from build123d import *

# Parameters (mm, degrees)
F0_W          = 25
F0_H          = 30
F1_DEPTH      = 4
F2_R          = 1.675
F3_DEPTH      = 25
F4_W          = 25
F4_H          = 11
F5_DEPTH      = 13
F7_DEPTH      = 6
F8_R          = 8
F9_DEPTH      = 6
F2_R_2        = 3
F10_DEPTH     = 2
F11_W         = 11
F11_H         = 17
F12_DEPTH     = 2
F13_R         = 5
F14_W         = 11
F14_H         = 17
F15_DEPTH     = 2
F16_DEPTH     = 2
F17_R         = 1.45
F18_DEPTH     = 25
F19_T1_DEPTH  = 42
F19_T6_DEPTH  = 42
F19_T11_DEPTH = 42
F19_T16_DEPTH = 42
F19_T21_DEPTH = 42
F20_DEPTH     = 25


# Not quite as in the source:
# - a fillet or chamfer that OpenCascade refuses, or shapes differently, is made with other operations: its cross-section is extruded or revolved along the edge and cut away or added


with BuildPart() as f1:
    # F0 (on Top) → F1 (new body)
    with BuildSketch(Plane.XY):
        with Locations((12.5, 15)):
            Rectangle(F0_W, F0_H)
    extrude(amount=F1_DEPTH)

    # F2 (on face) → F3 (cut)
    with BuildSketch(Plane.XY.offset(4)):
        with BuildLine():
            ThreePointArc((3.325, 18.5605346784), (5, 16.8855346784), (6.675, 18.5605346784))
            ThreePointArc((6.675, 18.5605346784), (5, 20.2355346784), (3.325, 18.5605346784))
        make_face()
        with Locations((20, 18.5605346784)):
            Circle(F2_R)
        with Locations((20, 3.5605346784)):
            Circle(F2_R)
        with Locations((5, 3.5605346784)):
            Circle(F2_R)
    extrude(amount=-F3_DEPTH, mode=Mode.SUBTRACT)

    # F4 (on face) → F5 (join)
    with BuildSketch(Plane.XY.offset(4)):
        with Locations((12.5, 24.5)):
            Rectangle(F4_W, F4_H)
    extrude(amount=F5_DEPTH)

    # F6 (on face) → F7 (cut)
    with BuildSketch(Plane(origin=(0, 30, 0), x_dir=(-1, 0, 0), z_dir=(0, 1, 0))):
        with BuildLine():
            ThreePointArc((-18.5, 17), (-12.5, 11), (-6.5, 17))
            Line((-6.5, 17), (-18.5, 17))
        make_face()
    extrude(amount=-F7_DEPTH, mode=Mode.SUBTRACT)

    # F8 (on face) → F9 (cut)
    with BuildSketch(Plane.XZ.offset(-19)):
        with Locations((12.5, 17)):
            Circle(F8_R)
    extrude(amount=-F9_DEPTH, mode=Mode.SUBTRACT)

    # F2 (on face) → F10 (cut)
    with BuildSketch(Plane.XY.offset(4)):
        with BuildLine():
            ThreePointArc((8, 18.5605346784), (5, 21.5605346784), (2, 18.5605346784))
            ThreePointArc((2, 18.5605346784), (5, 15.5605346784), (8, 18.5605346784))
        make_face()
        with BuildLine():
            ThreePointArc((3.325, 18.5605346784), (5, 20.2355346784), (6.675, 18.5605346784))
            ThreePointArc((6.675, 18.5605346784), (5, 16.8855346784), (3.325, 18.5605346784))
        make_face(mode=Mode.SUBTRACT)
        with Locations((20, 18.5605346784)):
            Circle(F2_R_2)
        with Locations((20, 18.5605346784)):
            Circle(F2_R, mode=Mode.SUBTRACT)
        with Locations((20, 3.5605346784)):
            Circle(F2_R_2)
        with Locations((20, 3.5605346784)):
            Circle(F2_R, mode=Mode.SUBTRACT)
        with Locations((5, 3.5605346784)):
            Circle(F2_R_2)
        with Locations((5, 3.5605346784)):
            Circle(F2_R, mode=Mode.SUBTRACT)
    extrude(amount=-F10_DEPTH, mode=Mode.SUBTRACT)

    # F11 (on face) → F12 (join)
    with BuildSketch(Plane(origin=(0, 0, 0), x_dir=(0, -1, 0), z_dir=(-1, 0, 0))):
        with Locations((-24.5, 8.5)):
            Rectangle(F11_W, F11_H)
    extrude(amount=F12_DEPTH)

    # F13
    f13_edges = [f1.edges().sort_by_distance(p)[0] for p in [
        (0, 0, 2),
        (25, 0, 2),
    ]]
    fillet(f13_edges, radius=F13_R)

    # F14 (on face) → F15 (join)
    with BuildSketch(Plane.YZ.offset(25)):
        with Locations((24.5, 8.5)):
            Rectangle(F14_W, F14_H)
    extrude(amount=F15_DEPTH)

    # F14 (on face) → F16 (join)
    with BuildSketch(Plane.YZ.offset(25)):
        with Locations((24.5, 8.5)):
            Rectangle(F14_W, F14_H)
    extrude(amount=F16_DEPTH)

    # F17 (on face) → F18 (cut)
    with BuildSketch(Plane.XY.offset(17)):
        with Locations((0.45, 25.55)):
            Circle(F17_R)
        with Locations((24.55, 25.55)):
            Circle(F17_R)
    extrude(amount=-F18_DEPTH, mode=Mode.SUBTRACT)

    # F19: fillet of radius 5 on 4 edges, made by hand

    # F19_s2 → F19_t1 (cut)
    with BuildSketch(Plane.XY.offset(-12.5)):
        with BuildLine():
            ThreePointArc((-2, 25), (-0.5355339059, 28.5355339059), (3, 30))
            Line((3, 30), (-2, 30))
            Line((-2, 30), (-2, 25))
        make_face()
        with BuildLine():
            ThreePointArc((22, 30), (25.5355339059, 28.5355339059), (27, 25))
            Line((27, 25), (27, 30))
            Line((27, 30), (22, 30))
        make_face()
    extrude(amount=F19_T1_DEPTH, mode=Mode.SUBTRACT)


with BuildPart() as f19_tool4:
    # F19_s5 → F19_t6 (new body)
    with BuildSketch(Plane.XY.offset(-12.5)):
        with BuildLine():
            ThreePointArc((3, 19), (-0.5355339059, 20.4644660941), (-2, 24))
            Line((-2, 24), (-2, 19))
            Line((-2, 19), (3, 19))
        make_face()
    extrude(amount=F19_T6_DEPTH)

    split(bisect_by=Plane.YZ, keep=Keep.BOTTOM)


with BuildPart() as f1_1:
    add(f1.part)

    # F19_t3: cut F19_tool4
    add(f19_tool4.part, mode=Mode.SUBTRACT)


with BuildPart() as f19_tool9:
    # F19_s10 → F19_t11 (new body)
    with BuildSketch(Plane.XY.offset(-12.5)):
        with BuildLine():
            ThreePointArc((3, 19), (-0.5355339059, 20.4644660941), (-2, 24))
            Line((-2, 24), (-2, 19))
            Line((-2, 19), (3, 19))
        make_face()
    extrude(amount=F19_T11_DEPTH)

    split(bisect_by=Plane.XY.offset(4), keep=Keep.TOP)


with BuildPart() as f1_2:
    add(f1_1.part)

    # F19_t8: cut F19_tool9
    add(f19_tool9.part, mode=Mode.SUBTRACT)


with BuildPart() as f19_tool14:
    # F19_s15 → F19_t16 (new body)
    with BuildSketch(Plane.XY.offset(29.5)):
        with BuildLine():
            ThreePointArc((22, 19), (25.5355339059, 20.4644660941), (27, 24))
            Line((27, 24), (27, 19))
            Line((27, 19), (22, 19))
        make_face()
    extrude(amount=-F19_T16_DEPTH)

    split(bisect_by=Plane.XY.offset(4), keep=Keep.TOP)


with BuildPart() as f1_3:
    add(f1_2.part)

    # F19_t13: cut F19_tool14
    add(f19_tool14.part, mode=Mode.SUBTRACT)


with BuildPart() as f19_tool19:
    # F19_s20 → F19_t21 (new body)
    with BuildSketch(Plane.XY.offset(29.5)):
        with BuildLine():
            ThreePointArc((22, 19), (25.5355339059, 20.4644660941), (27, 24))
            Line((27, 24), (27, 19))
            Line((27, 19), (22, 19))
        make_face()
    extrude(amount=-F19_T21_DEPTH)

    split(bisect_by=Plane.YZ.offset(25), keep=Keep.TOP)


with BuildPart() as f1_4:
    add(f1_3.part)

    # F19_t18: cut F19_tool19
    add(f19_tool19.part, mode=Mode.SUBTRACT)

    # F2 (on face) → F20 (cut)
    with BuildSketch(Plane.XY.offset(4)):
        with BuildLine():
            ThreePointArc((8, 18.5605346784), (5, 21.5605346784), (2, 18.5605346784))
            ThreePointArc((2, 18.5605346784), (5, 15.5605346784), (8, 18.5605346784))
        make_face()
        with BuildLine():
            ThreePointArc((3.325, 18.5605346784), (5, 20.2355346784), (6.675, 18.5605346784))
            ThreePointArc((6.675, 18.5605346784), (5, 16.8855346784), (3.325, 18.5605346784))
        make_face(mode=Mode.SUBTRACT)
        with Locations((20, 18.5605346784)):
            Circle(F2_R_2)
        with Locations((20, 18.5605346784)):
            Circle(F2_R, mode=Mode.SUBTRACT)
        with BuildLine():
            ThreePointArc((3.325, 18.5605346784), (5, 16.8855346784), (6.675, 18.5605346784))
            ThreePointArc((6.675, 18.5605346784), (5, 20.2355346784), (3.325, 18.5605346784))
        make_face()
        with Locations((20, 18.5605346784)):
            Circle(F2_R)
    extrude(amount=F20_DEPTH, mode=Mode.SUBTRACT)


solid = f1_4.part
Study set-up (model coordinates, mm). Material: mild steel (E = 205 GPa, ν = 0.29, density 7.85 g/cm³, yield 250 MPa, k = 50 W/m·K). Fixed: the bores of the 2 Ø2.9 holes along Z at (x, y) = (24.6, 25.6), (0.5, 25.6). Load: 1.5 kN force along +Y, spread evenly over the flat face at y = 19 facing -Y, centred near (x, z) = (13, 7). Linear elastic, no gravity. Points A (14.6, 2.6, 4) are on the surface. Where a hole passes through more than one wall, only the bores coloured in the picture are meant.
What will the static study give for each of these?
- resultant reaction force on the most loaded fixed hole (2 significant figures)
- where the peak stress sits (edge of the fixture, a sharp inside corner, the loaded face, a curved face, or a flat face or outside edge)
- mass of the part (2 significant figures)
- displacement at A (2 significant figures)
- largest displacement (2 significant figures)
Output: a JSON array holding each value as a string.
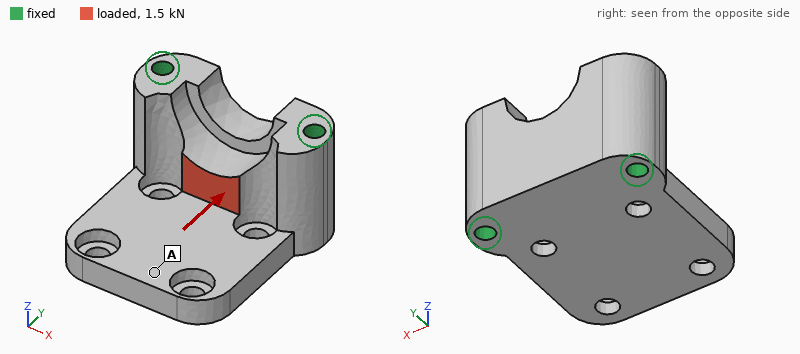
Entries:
["770 N", "a curved face", "41 g", "2.2 µm", "2.5 µm"]
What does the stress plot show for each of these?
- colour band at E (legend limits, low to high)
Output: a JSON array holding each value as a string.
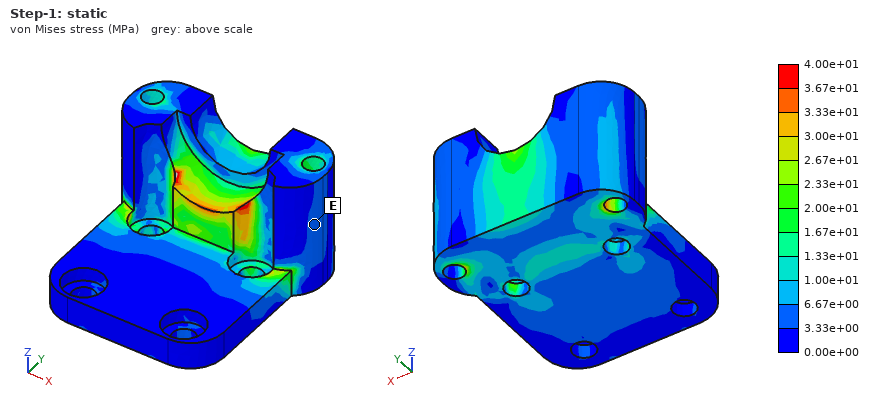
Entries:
["3.33e+00 to 6.67e+00 MPa"]
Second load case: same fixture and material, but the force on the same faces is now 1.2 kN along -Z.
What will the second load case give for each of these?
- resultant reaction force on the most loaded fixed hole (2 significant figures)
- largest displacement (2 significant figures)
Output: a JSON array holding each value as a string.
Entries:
["620 N", "4.9 µm"]
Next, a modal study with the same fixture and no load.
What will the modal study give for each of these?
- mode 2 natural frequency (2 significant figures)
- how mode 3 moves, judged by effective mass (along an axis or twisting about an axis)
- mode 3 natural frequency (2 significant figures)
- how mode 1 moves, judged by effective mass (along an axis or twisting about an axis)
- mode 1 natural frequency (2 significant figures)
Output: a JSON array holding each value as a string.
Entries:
["15 kHz", "along X", "23 kHz", "along Z", "6800 Hz"]
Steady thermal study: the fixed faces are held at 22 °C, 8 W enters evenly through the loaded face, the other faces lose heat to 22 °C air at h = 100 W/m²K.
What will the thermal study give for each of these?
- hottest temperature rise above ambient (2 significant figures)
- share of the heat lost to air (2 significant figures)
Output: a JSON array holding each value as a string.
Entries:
["16 K", "11 %"]
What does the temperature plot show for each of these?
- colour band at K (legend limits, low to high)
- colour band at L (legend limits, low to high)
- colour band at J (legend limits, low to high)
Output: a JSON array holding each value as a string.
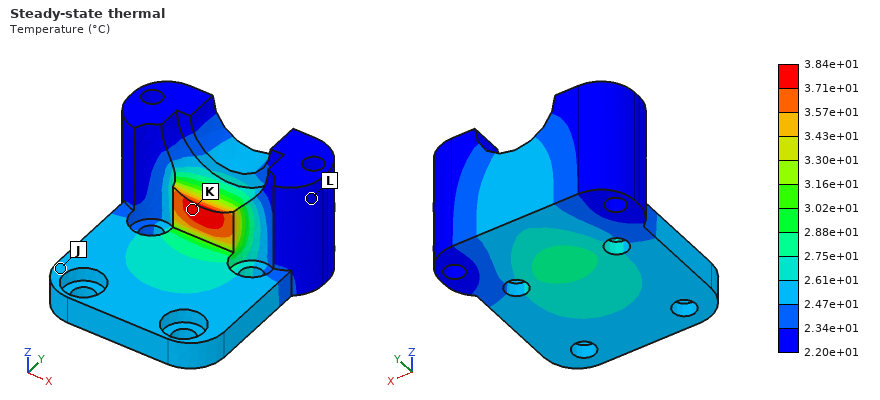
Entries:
["3.71e+01 to 3.84e+01 °C", "2.20e+01 to 2.34e+01 °C", "2.47e+01 to 2.61e+01 °C"]
